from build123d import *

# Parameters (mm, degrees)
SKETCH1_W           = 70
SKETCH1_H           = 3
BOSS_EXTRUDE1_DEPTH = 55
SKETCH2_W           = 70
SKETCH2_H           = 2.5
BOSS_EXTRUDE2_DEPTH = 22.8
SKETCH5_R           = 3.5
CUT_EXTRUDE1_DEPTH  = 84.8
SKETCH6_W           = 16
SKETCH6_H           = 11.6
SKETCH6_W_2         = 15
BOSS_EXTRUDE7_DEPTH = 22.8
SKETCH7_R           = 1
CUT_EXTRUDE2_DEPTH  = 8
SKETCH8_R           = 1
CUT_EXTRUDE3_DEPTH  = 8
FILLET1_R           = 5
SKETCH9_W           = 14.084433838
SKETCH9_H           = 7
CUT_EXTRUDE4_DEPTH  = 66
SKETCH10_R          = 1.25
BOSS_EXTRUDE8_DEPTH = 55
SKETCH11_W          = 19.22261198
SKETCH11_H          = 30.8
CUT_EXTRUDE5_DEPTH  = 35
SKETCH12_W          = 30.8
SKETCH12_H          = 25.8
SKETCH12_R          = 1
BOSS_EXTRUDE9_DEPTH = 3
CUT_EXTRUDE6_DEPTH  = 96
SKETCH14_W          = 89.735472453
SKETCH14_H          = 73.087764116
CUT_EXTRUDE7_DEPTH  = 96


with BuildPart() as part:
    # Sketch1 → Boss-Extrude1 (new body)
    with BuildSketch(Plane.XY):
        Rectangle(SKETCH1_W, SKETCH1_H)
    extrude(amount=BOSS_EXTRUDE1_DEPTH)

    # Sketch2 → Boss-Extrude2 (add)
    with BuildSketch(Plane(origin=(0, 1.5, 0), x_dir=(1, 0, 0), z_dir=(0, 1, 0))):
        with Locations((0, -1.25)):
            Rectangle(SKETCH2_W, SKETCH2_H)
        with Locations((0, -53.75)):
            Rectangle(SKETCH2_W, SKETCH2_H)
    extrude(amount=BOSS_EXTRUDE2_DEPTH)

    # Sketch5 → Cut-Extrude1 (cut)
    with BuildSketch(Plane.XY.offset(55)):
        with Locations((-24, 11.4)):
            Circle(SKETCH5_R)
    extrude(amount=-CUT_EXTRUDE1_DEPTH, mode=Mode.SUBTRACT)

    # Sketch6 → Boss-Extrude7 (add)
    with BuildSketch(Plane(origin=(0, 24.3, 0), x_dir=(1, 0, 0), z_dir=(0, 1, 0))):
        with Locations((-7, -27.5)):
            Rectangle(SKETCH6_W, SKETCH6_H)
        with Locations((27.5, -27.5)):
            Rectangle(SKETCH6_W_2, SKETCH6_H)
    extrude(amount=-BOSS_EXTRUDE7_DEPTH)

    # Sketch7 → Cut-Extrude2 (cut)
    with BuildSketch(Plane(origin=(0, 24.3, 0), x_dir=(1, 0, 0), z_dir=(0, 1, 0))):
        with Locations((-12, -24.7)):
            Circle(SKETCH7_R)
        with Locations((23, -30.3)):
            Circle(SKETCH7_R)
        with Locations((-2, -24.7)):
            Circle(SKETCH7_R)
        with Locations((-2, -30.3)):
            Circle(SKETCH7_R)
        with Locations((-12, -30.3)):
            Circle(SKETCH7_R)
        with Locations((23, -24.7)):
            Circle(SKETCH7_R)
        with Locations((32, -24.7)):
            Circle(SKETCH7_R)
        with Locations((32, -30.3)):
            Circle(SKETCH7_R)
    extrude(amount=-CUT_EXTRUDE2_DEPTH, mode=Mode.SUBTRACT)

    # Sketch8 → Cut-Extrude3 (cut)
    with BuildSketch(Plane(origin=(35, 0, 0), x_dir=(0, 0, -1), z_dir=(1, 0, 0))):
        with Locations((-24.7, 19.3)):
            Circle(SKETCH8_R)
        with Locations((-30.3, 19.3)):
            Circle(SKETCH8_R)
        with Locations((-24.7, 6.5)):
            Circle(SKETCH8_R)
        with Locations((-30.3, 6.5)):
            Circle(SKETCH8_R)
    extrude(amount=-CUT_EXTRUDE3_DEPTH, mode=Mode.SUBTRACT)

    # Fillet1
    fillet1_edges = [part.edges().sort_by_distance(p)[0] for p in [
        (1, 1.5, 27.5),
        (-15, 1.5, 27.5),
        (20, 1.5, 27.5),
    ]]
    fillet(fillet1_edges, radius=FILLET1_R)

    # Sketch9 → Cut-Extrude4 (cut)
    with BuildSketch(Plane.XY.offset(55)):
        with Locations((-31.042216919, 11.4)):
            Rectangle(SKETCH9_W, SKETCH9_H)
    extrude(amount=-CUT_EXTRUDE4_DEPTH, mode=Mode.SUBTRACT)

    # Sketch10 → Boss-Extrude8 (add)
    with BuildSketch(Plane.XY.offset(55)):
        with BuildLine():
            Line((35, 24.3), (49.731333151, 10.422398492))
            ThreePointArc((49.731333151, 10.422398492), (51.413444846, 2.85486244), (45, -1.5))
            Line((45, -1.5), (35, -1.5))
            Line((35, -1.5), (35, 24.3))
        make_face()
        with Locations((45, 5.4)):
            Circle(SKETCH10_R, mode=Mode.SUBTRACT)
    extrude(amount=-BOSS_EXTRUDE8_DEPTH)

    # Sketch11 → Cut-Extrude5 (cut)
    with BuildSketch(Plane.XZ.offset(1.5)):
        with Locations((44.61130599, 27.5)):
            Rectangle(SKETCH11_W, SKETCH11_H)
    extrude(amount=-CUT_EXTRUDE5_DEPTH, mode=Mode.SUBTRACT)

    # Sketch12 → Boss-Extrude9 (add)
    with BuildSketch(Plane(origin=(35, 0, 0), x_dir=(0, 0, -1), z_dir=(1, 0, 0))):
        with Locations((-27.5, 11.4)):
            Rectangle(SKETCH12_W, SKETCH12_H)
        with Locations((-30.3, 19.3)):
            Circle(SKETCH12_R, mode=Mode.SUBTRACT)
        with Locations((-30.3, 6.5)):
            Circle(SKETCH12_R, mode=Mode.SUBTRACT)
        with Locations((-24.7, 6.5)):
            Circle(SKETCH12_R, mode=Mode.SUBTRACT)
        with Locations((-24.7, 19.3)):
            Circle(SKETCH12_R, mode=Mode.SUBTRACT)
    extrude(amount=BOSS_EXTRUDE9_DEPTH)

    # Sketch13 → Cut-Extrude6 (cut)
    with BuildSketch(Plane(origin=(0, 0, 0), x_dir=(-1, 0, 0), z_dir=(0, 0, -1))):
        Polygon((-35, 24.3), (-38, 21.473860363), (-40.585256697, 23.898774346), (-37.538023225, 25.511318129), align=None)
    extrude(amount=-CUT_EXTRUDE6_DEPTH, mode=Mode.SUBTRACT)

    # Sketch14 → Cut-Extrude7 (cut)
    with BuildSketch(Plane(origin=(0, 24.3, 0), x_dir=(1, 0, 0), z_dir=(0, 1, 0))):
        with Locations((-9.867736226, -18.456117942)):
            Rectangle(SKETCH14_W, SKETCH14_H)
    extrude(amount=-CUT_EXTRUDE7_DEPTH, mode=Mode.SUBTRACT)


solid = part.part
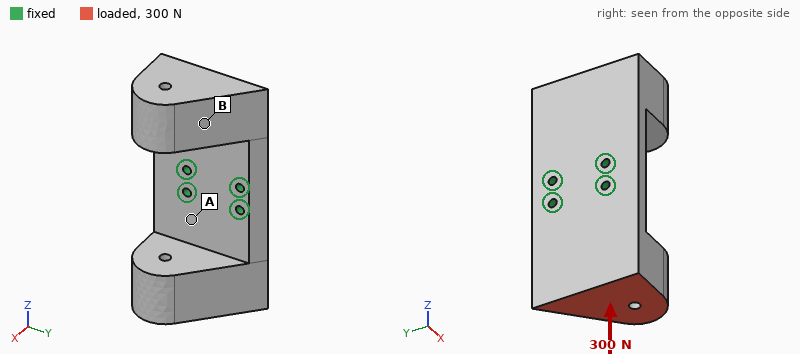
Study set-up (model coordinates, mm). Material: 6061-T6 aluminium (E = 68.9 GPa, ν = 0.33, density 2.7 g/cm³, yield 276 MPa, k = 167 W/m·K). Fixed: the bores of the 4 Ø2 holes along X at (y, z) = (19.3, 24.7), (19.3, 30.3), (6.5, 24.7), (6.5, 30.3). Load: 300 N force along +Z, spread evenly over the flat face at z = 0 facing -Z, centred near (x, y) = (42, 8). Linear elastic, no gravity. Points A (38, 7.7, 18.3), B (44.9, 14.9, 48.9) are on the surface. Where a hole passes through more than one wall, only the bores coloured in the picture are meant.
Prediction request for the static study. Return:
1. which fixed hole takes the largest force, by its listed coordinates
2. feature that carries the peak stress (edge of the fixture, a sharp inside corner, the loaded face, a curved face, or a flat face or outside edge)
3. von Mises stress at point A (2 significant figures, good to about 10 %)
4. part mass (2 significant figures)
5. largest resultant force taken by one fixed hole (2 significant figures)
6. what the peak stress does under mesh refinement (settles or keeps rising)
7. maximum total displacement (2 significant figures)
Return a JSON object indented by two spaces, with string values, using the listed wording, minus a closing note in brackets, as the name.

{
  "which fixed hole takes the largest force, by its listed coordinates": "(6.5, 24.7)",
  "feature that carries the peak stress": "edge of the fixture",
  "von Mises stress at point A": "45 MPa",
  "part mass": "25 g",
  "largest resultant force taken by one fixed hole": "180 N",
  "what the peak stress does under mesh refinement": "keeps rising",
  "maximum total displacement": "0.14 mm"
}
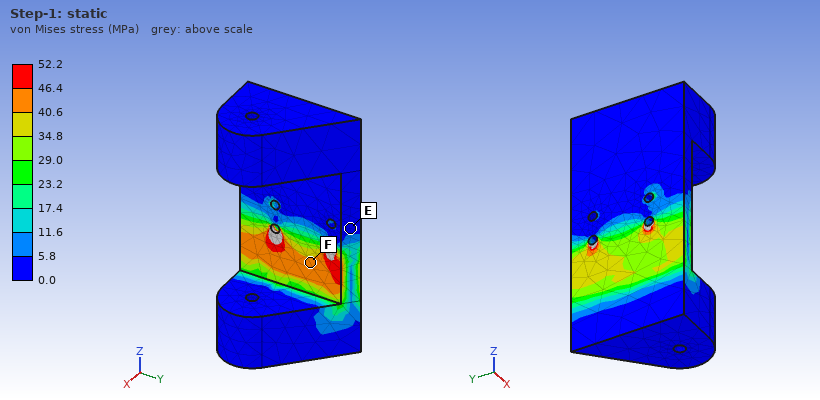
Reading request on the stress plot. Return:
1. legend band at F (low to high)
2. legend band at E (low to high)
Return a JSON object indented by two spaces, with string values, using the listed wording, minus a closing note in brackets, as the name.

{
  "legend band at F": "40.6 to 46.4 MPa",
  "legend band at E": "0.0 to 5.8 MPa"
}
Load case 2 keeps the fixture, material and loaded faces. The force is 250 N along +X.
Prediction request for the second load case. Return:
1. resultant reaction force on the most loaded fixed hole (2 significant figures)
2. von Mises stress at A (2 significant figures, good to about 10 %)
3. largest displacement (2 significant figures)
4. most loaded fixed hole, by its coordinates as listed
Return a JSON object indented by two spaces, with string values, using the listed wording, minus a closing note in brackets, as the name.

{
  "resultant reaction force on the most loaded fixed hole": "460 N",
  "von Mises stress at A": "110 MPa",
  "largest displacement": "0.41 mm",
  "most loaded fixed hole, by its coordinates as listed": "(6.5, 24.7)"
}
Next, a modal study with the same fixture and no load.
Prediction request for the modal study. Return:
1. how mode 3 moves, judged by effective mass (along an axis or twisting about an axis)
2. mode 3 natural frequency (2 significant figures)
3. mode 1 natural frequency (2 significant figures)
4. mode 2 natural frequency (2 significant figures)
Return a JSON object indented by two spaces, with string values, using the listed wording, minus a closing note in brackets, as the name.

{
  "how mode 3 moves, judged by effective mass": "twisting about X",
  "mode 3 natural frequency": "4900 Hz",
  "mode 1 natural frequency": "1800 Hz",
  "mode 2 natural frequency": "1800 Hz"
}
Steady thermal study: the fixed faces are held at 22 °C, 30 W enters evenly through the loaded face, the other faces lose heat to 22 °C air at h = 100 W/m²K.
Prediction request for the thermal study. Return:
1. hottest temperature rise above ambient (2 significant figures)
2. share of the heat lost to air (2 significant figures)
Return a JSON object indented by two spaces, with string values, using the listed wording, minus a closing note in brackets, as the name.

{
  "hottest temperature rise above ambient": "42 K",
  "share of the heat lost to air": "18 %"
}
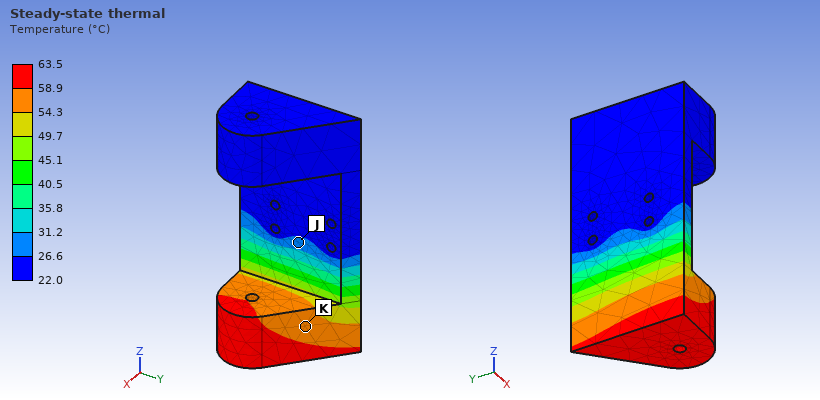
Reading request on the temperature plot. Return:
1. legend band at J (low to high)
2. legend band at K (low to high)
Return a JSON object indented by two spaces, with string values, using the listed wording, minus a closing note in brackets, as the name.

{
  "legend band at J": "26.6 to 31.2 °C",
  "legend band at K": "54.3 to 58.9 °C"
}
